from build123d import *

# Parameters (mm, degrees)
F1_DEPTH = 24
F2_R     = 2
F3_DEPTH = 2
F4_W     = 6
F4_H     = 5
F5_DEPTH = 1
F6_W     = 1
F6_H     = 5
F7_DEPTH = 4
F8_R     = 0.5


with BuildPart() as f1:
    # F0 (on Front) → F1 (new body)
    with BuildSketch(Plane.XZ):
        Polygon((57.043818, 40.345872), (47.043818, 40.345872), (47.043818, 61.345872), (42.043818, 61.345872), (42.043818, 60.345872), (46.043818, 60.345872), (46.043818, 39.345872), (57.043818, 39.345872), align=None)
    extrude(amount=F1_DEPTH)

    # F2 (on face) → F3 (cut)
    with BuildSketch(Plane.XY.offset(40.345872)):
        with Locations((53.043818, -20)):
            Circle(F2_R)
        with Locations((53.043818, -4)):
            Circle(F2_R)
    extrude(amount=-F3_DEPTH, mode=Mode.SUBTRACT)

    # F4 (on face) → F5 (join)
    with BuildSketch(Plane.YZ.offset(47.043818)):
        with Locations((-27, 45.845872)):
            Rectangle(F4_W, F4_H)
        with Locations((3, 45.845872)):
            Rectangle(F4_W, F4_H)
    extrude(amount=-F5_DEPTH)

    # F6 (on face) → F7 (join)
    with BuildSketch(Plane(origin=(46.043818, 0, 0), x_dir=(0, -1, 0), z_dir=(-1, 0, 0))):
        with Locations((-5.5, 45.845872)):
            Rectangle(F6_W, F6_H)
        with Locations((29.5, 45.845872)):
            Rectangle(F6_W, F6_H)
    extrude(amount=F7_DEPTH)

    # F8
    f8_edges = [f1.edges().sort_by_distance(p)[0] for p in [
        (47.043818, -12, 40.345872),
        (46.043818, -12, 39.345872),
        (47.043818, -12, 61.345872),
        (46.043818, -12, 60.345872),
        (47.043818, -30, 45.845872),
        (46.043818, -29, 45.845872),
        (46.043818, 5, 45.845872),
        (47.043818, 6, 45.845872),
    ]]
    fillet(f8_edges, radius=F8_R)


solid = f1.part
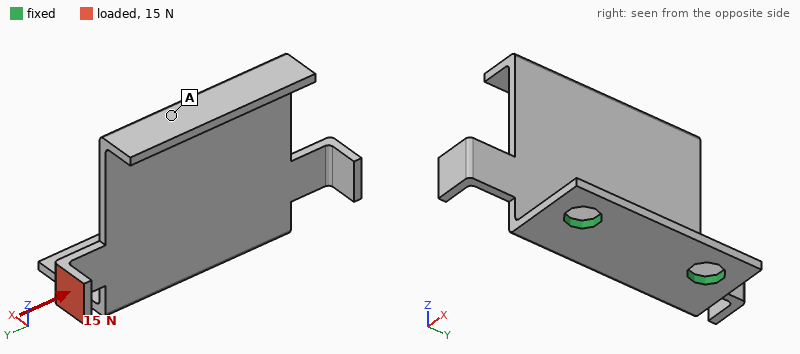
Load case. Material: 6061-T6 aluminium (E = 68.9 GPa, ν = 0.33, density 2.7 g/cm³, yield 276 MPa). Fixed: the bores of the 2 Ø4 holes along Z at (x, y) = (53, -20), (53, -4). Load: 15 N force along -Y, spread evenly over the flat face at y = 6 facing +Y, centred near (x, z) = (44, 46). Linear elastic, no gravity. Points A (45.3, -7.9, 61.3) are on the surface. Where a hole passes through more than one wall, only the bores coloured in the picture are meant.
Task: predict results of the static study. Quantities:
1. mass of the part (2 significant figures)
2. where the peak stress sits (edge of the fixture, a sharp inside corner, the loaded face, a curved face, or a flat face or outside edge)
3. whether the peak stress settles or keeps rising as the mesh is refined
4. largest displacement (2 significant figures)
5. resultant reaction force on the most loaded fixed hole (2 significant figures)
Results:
2.5 g
a sharp inside corner
keeps rising
64 µm
12 N
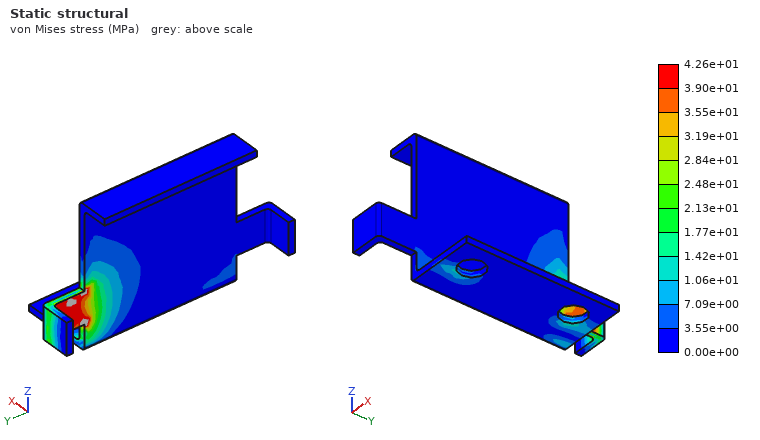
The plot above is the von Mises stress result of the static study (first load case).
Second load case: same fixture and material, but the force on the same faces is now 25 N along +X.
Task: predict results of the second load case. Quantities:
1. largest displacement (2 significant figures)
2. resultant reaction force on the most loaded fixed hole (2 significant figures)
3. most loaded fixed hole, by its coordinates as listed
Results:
0.40 mm
37 N
(53, -4)
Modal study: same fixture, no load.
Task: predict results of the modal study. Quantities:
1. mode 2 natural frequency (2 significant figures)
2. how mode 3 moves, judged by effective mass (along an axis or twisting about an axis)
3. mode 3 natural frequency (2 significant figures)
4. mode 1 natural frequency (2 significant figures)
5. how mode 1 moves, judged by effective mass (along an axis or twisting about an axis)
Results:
2700 Hz
along Y
4200 Hz
1000 Hz
along X
